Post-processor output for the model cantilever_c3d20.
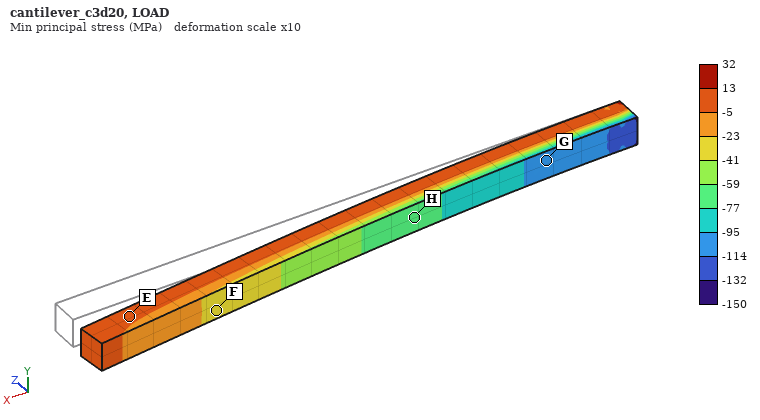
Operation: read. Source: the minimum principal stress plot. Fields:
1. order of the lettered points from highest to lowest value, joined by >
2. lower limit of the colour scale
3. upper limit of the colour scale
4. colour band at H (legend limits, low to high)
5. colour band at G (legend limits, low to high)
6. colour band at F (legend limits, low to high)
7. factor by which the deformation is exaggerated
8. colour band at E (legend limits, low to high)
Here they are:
E > F > H > G
-150 MPa
32 MPa
-77 to -59 MPa
-114 to -95 MPa
-41 to -23 MPa
10
-5 to 13 MPa
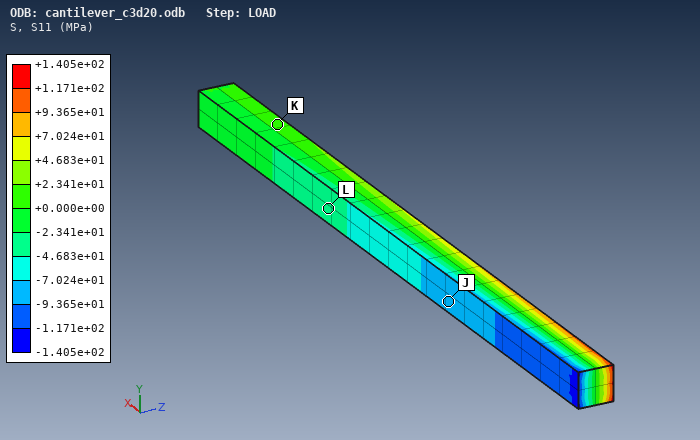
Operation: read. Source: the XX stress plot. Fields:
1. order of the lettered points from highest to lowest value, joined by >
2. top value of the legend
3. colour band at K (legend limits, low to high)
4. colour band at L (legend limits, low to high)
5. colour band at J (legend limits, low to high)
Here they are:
K > L > J
+1.405e+02 MPa
+0.000e+00 to +2.341e+01 MPa
-4.683e+01 to -2.341e+01 MPa
-9.365e+01 to -7.024e+01 MPa
